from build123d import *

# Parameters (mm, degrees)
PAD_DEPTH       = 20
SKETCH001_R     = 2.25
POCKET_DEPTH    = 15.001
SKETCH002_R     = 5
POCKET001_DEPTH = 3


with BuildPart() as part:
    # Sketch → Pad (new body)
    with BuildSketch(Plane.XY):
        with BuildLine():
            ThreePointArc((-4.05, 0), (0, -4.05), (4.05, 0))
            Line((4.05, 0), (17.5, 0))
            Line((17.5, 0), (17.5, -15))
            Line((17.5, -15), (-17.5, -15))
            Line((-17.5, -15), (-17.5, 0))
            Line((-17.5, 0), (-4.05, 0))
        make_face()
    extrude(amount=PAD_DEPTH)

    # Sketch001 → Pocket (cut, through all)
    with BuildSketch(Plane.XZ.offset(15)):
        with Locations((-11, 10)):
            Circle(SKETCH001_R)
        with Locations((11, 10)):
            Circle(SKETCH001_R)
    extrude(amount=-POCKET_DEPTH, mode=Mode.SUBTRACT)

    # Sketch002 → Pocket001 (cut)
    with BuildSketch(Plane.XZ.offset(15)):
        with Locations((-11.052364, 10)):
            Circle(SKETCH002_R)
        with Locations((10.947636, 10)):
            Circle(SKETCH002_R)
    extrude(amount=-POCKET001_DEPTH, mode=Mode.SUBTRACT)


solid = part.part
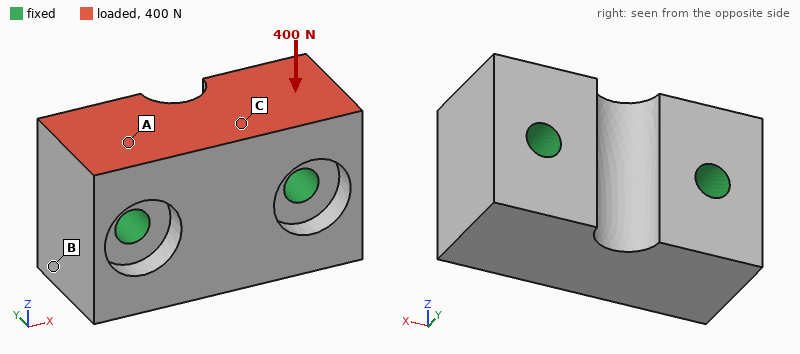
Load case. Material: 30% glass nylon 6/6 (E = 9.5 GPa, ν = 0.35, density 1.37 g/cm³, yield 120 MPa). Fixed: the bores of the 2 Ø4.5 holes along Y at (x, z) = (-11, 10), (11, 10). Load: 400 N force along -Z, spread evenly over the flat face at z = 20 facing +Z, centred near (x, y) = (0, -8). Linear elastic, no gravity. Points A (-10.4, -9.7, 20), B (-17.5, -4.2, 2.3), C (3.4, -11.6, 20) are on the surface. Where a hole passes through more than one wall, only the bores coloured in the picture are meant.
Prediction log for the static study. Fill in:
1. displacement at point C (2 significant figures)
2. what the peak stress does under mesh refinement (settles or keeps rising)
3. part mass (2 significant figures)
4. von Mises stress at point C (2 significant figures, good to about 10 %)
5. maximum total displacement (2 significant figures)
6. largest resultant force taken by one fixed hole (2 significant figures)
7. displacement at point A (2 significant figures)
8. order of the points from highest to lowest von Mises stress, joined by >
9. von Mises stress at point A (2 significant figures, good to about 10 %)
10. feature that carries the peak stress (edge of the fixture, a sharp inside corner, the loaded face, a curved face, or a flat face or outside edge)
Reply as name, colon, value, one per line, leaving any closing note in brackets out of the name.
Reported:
displacement at point C: 2.2 µm
what the peak stress does under mesh refinement: keeps rising
part mass: 13 g
von Mises stress at point C: 0.79 MPa
maximum total displacement: 2.6 µm
largest resultant force taken by one fixed hole: 200 N
displacement at point A: 1.5 µm
order of the points from highest to lowest von Mises stress, joined by >: A > C > B
von Mises stress at point A: 1.3 MPa
feature that carries the peak stress: edge of the fixture
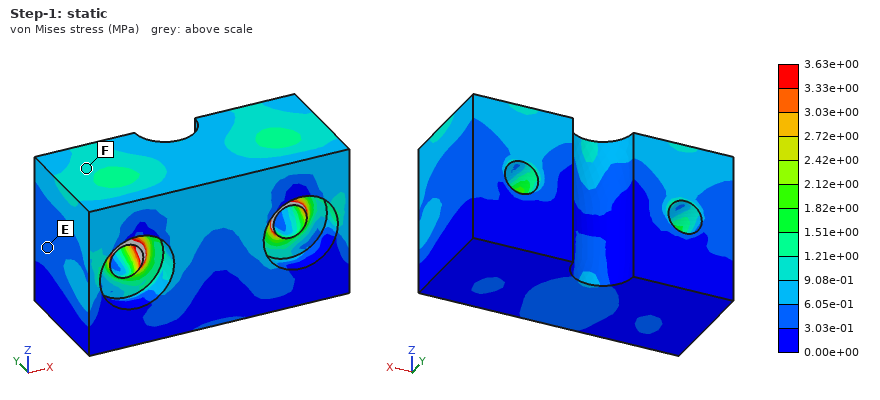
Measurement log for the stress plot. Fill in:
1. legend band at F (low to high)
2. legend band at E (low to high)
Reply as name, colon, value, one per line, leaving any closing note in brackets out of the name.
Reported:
legend band at F: 9.08e-01 to 1.21e+00 MPa
legend band at E: 3.03e-01 to 6.05e-01 MPa
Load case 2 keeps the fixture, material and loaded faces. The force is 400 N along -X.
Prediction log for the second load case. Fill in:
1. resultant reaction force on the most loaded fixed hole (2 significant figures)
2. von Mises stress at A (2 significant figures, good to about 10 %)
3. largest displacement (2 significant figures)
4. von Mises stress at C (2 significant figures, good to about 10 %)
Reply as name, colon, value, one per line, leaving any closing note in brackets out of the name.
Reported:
resultant reaction force on the most loaded fixed hole: 240 N
von Mises stress at A: 1.9 MPa
largest displacement: 5.7 µm
von Mises stress at C: 1.6 MPa
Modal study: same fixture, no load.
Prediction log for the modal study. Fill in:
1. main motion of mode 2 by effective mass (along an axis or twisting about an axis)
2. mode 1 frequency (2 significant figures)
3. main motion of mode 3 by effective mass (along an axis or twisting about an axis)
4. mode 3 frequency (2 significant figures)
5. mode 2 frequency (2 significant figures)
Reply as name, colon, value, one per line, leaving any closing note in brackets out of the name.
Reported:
main motion of mode 2 by effective mass: along Y
mode 1 frequency: 20 kHz
main motion of mode 3 by effective mass: twisting about Y
mode 3 frequency: 27 kHz
mode 2 frequency: 25 kHz
